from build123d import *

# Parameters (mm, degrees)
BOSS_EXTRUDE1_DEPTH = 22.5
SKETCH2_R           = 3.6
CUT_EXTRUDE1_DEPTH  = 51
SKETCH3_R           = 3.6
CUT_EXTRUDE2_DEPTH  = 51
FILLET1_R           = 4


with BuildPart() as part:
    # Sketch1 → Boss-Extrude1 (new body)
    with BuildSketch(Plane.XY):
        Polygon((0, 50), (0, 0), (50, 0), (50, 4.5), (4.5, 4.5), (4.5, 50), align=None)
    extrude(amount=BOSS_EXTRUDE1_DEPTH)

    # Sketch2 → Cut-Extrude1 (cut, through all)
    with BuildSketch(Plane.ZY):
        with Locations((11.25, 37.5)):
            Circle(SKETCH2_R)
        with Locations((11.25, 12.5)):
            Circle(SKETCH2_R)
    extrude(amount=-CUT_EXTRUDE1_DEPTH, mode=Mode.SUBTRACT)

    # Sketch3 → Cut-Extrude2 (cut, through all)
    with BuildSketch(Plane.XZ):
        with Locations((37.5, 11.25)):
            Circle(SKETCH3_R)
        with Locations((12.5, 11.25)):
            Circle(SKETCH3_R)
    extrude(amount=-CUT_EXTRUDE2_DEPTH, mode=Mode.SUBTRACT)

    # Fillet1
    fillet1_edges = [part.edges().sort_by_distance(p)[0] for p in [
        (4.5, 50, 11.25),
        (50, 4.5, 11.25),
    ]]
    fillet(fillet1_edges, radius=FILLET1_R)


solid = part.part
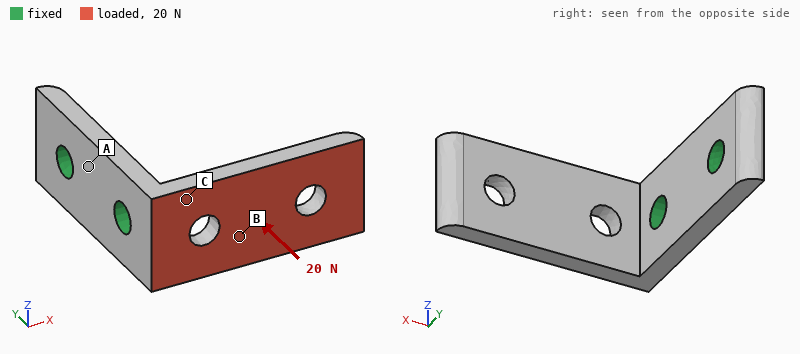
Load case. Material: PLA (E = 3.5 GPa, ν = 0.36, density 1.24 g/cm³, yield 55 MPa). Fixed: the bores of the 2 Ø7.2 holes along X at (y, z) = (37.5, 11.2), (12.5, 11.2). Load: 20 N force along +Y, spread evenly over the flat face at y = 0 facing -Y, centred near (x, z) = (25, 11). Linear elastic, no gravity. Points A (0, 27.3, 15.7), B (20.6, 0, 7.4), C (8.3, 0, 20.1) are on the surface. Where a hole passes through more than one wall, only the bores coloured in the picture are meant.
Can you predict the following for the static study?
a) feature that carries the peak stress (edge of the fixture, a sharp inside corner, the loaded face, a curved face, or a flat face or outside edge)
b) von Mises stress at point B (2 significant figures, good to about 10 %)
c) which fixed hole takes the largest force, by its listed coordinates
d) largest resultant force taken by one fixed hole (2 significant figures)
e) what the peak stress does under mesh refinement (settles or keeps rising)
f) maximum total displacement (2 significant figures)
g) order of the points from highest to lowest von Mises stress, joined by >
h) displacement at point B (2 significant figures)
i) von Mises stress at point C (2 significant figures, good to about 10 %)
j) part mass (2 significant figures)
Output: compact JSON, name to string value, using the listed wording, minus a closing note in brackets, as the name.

{"feature that carries the peak stress": "edge of the fixture", "von Mises stress at point B": "2.2 MPa", "which fixed hole takes the largest force, by its listed coordinates": "(12.5, 11.2)", "largest resultant force taken by one fixed hole": "19 N", "what the peak stress does under mesh refinement": "keeps rising", "maximum total displacement": "0.74 mm", "order of the points from highest to lowest von Mises stress, joined by >": "C > B > A", "displacement at point B": "0.21 mm", "von Mises stress at point C": "5.5 MPa", "part mass": "11 g"}
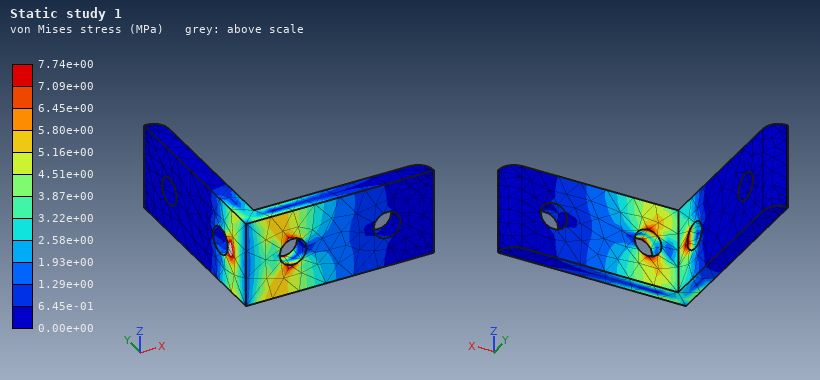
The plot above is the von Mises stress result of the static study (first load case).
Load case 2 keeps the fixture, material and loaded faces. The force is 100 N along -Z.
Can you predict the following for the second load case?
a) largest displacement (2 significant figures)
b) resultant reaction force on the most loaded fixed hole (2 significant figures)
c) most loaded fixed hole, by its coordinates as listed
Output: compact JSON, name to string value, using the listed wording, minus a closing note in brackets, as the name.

{"largest displacement": "0.80 mm", "resultant reaction force on the most loaded fixed hole": "120 N", "most loaded fixed hole, by its coordinates as listed": "(12.5, 11.2)"}
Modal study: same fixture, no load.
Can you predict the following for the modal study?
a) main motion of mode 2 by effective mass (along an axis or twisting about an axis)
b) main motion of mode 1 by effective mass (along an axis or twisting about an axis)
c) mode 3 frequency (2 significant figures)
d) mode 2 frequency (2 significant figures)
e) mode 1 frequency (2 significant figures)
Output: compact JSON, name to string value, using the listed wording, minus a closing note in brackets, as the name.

{"main motion of mode 2 by effective mass": "along Z", "main motion of mode 1 by effective mass": "along Y", "mode 3 frequency": "2000 Hz", "mode 2 frequency": "890 Hz", "mode 1 frequency": "440 Hz"}
